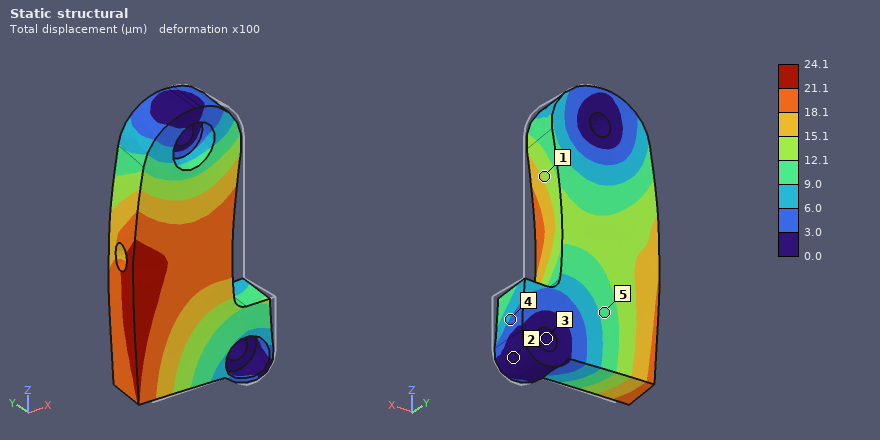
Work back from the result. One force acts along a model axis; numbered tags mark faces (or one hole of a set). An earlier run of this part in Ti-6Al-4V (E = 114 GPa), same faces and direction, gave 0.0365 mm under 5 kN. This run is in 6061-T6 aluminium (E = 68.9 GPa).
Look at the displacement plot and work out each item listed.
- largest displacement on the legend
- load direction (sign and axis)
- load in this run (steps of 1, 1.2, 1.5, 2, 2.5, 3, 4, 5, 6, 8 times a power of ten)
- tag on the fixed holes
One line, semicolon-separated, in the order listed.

24.1 µm; -X; 2 kN; 3
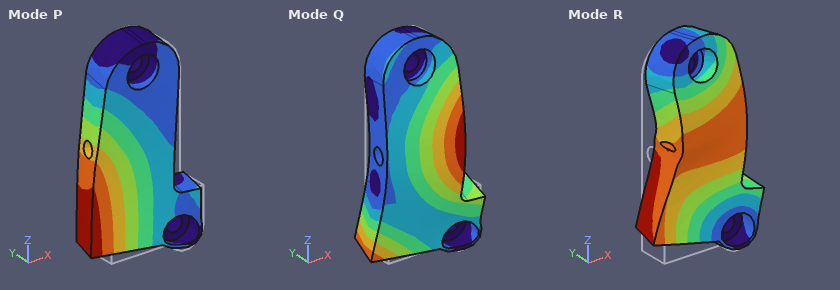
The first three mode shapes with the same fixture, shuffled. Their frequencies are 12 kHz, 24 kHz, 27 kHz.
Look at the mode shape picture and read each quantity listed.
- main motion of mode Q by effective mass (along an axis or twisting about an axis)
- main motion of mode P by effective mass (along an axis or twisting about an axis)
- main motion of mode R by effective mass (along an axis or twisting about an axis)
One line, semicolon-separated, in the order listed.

along Y; along Y; along X
